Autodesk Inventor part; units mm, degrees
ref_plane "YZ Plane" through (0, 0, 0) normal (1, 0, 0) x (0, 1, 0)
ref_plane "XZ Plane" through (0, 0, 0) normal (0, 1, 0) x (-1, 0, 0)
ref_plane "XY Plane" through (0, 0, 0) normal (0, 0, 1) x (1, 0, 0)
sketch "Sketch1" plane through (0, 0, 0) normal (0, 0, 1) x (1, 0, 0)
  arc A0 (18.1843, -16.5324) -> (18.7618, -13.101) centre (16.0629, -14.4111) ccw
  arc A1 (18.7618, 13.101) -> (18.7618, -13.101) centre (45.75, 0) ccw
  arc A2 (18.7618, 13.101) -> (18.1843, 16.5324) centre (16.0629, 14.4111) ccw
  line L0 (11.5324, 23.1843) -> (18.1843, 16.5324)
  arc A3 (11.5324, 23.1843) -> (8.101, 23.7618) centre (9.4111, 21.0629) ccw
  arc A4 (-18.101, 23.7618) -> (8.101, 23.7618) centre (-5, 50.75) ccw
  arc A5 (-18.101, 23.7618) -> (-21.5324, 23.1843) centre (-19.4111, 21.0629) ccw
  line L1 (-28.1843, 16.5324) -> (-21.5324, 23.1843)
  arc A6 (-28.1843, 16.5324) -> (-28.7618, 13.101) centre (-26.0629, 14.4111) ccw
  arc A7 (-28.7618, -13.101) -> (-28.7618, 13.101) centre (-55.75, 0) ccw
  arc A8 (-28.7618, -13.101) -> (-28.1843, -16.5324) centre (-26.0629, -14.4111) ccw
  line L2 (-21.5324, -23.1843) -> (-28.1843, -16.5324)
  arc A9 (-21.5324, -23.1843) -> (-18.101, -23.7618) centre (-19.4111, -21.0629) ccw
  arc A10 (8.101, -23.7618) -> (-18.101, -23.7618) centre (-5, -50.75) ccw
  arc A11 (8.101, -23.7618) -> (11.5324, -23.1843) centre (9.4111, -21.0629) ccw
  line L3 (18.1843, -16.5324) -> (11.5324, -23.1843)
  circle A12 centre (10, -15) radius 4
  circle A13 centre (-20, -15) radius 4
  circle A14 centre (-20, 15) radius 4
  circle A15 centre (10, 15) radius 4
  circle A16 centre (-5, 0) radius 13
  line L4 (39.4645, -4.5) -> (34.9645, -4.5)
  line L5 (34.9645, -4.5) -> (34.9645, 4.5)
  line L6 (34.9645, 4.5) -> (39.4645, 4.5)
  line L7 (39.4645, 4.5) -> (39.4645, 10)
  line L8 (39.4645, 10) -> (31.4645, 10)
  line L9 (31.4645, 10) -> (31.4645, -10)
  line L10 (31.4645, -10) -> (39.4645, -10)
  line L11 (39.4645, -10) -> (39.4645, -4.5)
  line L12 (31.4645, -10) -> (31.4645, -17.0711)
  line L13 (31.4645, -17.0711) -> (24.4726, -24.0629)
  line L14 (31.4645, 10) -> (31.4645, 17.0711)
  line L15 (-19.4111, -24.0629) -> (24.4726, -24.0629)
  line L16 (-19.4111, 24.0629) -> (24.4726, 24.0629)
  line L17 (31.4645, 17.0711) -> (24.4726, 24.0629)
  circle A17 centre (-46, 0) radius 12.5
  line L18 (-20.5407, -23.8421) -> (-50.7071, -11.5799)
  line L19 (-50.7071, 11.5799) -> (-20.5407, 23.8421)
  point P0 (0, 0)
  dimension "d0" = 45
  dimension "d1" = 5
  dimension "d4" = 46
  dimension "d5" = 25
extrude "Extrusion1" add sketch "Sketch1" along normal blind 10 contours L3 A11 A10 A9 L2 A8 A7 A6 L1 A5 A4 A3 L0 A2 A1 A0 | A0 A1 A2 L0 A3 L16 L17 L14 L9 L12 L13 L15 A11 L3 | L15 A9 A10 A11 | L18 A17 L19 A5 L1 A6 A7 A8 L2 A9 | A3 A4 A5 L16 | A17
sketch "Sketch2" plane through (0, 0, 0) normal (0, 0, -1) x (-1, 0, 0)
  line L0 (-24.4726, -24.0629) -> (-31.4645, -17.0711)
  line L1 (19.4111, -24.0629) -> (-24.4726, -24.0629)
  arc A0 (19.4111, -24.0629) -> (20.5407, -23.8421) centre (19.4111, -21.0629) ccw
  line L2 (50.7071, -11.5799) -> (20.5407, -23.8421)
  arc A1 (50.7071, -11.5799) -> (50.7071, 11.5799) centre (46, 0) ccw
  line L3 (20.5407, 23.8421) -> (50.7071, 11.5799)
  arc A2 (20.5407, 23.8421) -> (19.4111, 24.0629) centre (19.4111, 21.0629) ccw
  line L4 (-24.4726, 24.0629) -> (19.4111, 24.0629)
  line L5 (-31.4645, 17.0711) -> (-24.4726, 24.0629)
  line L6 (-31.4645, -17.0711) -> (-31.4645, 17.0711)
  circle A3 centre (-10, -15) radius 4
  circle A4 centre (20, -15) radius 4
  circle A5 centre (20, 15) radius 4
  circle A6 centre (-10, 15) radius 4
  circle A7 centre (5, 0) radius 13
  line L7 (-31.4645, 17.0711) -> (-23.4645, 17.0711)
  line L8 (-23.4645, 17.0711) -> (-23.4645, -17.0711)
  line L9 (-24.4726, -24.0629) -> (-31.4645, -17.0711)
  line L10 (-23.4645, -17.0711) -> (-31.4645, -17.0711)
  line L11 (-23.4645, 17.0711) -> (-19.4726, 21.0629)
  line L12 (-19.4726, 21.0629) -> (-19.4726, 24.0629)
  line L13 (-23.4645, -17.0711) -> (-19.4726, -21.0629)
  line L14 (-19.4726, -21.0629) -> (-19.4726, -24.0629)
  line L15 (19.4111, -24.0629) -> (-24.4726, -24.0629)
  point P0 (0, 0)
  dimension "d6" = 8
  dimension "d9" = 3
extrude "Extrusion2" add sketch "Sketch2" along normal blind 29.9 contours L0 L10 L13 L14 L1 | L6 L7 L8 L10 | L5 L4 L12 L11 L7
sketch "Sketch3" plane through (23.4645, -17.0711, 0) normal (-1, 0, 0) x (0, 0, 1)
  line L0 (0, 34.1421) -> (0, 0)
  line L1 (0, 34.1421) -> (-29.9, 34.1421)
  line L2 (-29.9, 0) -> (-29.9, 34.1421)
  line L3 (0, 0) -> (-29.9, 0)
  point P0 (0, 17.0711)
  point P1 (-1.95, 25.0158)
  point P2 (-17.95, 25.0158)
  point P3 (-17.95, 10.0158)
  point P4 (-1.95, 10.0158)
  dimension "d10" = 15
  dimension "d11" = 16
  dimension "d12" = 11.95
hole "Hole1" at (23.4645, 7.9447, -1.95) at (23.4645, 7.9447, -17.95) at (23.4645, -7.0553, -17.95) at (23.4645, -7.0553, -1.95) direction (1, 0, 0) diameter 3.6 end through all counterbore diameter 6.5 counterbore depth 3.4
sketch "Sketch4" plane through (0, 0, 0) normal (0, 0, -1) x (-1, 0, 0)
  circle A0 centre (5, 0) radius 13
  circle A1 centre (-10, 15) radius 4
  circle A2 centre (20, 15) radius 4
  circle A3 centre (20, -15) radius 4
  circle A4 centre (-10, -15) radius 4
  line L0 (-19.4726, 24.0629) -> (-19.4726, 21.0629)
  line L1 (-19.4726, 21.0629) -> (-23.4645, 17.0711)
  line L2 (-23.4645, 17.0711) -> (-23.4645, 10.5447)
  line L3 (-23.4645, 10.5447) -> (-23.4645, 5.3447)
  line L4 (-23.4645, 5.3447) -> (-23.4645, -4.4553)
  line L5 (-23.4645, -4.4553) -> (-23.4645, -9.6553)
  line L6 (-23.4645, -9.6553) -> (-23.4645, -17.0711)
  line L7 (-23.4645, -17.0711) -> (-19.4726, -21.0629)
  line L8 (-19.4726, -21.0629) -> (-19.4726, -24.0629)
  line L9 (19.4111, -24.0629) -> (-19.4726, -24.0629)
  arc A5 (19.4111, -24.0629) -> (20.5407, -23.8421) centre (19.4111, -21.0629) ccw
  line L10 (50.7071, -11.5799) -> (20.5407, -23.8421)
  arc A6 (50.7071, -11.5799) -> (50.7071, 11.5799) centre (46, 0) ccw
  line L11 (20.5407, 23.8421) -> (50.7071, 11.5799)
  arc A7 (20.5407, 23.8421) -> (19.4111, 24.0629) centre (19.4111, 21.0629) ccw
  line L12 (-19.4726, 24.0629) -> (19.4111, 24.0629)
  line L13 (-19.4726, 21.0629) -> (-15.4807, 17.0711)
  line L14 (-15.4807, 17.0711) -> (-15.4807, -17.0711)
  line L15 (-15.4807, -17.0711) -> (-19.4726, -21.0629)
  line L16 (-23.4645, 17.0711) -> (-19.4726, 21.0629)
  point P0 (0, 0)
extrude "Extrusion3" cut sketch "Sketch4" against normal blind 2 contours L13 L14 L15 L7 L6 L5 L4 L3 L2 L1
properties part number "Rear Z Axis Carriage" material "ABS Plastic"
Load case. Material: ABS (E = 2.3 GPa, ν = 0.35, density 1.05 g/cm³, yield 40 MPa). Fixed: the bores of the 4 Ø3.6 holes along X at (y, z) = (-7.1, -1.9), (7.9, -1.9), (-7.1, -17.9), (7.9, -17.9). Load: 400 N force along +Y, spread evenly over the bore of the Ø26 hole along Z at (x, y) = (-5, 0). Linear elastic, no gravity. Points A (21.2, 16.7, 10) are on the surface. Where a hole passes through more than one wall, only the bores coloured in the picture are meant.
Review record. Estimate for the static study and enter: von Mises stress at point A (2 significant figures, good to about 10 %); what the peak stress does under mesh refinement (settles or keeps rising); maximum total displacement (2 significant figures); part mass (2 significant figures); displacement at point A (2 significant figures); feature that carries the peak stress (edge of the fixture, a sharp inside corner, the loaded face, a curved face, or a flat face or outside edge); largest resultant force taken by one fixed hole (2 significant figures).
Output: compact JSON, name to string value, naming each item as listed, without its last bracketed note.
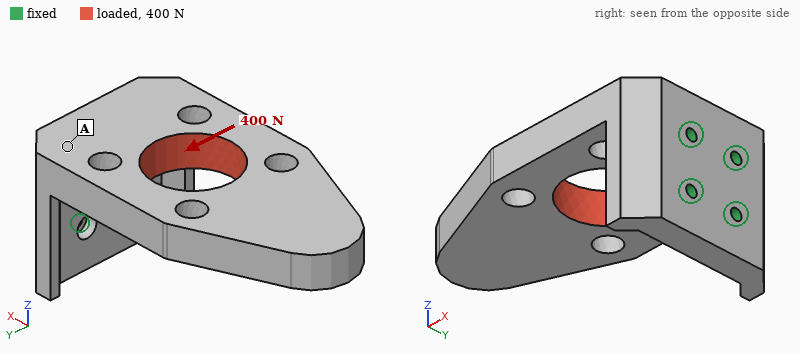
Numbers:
{"von Mises stress at point A": "3.7 MPa", "what the peak stress does under mesh refinement": "keeps rising", "maximum total displacement": "1.2 mm", "part mass": "41 g", "displacement at point A": "0.24 mm", "feature that carries the peak stress": "edge of the fixture", "largest resultant force taken by one fixed hole": "680 N"}
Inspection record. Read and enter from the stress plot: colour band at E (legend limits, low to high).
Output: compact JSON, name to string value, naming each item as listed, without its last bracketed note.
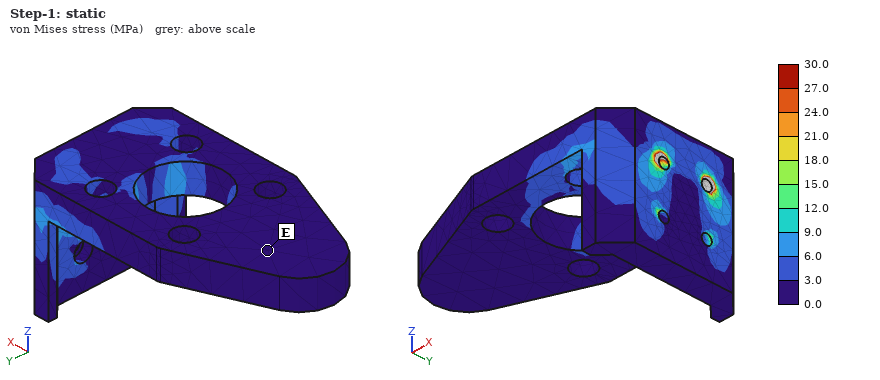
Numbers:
{"colour band at E": "0.0 to 3.0 MPa"}
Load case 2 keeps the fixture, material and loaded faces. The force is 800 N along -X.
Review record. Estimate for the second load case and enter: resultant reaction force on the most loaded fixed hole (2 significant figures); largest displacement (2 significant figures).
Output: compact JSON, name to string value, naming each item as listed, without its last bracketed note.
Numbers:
{"resultant reaction force on the most loaded fixed hole": "530 N", "largest displacement": "0.81 mm"}
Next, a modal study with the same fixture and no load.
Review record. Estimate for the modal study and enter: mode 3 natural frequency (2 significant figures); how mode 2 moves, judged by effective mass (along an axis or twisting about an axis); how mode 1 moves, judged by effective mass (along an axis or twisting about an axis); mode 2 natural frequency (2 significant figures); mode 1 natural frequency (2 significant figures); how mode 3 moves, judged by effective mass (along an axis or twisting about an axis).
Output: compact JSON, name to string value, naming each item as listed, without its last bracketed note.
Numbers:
{"mode 3 natural frequency": "1200 Hz", "how mode 2 moves, judged by effective mass": "along Y", "how mode 1 moves, judged by effective mass": "along Z", "mode 2 natural frequency": "580 Hz", "mode 1 natural frequency": "250 Hz", "how mode 3 moves, judged by effective mass": "twisting about X"}
